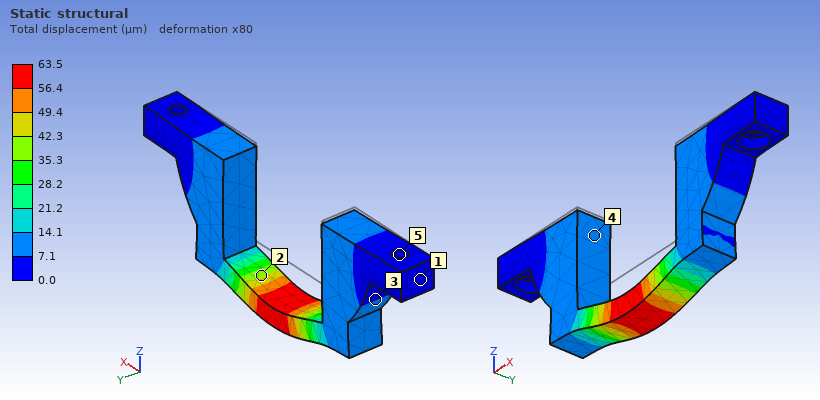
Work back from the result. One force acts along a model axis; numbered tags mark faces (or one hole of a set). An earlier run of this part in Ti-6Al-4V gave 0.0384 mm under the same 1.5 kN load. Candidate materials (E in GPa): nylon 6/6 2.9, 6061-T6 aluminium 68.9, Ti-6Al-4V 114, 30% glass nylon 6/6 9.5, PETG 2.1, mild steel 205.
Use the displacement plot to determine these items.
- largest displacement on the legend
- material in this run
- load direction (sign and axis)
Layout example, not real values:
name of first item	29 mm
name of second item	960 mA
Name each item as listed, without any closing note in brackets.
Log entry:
largest displacement on the legend	63.5 µm
material in this run	6061-T6 aluminium
load direction	-Z
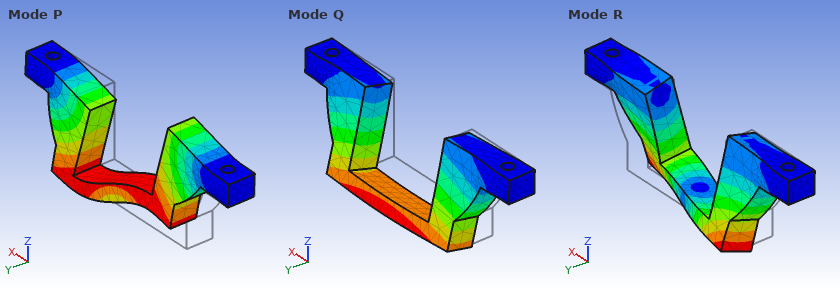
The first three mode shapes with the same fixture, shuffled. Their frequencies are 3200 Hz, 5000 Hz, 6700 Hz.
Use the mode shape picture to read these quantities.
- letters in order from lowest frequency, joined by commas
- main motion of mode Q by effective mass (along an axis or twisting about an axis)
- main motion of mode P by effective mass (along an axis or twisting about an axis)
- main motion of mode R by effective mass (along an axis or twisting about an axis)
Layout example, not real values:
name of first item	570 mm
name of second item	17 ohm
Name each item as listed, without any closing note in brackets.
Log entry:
letters in order from lowest frequency, joined by commas	Q, P, R
main motion of mode Q by effective mass	along Y
main motion of mode P by effective mass	along X
main motion of mode R by effective mass	twisting about Z
